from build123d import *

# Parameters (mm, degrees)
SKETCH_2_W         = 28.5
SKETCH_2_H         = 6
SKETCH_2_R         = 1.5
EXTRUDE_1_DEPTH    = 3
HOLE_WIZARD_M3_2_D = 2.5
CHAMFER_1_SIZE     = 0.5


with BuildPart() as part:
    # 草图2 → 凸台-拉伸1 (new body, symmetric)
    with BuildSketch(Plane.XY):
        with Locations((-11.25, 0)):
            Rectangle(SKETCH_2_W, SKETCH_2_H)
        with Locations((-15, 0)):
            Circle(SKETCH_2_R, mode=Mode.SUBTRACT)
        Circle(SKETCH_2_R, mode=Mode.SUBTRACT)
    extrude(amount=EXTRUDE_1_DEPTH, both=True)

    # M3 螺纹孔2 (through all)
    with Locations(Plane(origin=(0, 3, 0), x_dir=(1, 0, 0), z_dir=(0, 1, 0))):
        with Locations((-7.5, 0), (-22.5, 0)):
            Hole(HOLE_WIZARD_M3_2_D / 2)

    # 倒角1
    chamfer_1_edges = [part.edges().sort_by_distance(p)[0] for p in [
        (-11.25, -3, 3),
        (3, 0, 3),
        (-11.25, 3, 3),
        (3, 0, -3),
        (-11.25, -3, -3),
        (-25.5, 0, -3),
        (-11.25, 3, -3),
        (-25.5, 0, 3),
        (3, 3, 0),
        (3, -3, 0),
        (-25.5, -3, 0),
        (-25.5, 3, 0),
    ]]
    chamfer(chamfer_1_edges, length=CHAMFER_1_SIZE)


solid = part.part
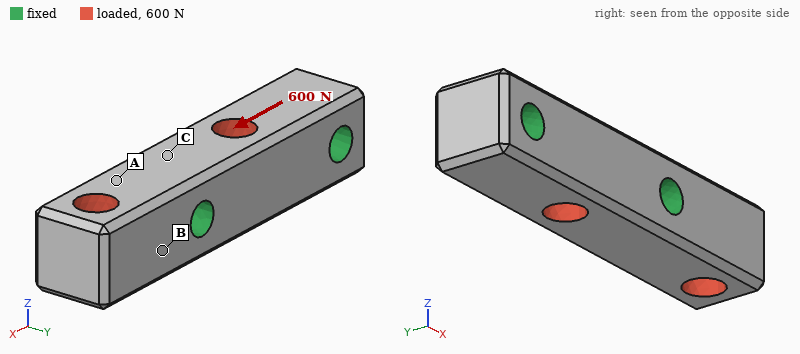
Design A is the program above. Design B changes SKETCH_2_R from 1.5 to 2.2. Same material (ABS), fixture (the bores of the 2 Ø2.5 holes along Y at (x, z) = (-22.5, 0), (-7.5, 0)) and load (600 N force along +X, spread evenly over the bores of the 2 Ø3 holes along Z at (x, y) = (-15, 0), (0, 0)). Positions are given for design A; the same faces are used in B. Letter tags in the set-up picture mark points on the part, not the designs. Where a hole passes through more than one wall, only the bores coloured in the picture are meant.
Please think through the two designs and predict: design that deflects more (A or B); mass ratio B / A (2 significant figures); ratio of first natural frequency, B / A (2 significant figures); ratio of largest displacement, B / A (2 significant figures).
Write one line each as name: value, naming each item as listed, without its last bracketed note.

design that deflects more: B
mass ratio B / A: 0.89
ratio of first natural frequency, B / A: 0.98
ratio of largest displacement, B / A: 2.5
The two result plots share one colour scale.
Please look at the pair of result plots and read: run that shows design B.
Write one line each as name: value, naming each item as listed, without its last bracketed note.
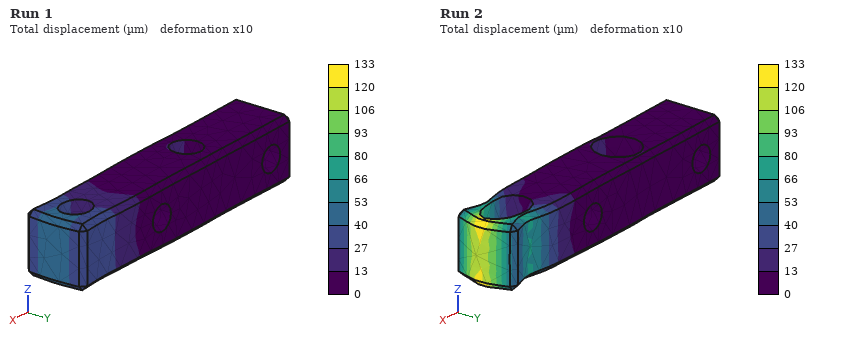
run that shows design B: Run 2
